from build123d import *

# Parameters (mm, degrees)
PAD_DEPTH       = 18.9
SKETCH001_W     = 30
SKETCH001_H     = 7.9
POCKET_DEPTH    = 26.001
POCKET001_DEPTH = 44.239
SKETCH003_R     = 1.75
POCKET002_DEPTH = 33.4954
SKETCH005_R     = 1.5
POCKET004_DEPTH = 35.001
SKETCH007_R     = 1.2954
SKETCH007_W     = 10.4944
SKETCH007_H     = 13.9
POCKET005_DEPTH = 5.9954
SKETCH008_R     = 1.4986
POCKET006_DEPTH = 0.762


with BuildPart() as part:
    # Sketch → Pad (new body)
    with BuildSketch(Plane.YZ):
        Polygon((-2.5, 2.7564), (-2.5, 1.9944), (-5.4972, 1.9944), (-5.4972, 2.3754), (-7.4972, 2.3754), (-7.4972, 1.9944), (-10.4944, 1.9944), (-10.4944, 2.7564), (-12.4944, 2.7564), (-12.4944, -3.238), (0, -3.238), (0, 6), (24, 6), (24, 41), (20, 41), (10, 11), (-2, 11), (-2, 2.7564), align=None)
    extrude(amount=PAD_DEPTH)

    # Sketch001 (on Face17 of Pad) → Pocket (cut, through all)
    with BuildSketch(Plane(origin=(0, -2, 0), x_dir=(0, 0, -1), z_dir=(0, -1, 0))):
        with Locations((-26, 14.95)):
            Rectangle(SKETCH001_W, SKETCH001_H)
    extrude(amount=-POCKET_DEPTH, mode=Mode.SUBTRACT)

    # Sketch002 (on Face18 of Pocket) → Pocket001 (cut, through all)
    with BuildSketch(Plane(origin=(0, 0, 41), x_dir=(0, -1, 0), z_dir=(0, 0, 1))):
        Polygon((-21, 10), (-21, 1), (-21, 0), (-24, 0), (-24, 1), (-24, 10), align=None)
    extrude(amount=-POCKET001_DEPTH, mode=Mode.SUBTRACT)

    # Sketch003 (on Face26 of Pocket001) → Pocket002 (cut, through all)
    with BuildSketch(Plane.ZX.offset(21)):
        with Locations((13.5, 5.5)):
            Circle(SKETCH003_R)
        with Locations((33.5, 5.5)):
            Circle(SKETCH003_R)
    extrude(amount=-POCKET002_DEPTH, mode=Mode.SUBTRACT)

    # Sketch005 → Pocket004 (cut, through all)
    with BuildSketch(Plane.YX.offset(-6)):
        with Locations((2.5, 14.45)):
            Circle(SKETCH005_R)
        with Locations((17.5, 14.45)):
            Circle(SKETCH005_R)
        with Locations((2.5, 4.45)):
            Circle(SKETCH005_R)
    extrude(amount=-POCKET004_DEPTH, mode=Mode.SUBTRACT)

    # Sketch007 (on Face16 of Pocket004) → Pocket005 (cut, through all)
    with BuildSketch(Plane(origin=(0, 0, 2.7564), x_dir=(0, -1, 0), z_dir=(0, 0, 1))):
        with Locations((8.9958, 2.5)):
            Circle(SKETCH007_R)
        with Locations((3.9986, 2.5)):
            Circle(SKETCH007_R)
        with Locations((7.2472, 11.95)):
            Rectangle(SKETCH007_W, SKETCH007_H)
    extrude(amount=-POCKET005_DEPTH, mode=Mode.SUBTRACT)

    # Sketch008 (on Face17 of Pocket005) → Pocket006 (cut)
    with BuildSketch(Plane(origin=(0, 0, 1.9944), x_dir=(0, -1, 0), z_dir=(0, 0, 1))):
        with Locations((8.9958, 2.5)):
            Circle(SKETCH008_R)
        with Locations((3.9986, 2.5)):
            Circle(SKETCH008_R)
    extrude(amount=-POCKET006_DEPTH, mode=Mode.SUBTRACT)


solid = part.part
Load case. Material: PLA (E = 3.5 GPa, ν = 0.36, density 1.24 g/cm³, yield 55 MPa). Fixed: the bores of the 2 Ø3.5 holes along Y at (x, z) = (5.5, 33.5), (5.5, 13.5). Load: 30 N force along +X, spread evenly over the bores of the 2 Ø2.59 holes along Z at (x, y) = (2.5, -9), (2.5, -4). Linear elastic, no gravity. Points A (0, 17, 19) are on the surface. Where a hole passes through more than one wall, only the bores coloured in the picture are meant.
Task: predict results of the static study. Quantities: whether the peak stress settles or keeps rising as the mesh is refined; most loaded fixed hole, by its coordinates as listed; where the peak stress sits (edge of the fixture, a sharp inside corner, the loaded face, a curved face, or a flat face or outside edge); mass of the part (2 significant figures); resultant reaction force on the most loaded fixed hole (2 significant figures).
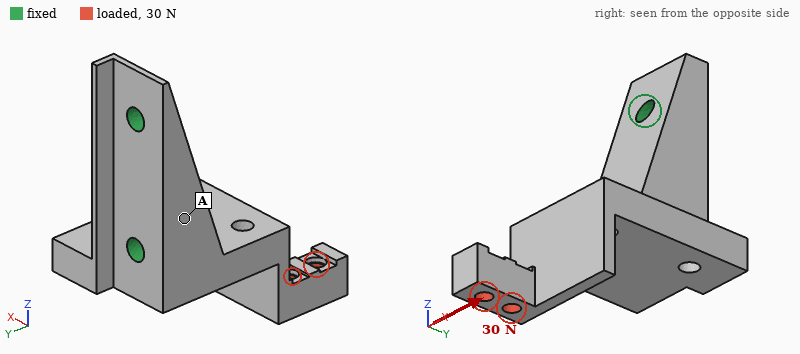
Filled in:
keeps rising
(5.5, 13.5)
a sharp inside corner
5.9 g
39 N
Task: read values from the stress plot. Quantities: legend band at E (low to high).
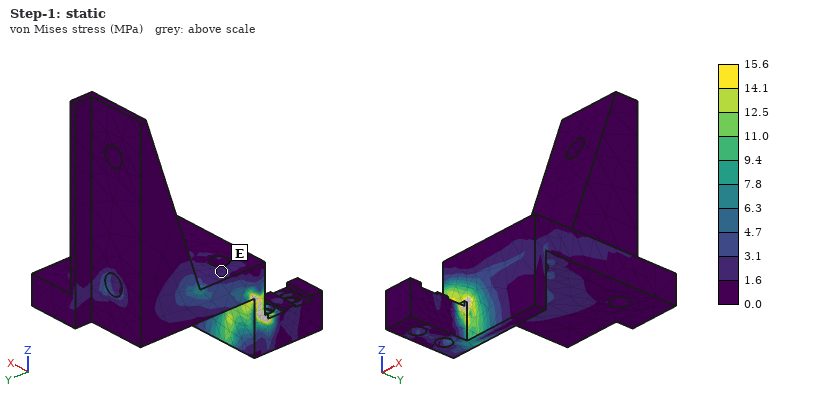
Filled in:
1.6 to 3.1 MPa
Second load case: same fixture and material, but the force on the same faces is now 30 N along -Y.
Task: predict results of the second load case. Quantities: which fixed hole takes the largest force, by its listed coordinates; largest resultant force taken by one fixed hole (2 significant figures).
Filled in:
(5.5, 13.5)
32 N
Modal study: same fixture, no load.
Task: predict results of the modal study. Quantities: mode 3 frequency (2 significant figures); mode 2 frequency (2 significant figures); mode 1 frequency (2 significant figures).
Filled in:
3700 Hz
2700 Hz
1700 Hz
